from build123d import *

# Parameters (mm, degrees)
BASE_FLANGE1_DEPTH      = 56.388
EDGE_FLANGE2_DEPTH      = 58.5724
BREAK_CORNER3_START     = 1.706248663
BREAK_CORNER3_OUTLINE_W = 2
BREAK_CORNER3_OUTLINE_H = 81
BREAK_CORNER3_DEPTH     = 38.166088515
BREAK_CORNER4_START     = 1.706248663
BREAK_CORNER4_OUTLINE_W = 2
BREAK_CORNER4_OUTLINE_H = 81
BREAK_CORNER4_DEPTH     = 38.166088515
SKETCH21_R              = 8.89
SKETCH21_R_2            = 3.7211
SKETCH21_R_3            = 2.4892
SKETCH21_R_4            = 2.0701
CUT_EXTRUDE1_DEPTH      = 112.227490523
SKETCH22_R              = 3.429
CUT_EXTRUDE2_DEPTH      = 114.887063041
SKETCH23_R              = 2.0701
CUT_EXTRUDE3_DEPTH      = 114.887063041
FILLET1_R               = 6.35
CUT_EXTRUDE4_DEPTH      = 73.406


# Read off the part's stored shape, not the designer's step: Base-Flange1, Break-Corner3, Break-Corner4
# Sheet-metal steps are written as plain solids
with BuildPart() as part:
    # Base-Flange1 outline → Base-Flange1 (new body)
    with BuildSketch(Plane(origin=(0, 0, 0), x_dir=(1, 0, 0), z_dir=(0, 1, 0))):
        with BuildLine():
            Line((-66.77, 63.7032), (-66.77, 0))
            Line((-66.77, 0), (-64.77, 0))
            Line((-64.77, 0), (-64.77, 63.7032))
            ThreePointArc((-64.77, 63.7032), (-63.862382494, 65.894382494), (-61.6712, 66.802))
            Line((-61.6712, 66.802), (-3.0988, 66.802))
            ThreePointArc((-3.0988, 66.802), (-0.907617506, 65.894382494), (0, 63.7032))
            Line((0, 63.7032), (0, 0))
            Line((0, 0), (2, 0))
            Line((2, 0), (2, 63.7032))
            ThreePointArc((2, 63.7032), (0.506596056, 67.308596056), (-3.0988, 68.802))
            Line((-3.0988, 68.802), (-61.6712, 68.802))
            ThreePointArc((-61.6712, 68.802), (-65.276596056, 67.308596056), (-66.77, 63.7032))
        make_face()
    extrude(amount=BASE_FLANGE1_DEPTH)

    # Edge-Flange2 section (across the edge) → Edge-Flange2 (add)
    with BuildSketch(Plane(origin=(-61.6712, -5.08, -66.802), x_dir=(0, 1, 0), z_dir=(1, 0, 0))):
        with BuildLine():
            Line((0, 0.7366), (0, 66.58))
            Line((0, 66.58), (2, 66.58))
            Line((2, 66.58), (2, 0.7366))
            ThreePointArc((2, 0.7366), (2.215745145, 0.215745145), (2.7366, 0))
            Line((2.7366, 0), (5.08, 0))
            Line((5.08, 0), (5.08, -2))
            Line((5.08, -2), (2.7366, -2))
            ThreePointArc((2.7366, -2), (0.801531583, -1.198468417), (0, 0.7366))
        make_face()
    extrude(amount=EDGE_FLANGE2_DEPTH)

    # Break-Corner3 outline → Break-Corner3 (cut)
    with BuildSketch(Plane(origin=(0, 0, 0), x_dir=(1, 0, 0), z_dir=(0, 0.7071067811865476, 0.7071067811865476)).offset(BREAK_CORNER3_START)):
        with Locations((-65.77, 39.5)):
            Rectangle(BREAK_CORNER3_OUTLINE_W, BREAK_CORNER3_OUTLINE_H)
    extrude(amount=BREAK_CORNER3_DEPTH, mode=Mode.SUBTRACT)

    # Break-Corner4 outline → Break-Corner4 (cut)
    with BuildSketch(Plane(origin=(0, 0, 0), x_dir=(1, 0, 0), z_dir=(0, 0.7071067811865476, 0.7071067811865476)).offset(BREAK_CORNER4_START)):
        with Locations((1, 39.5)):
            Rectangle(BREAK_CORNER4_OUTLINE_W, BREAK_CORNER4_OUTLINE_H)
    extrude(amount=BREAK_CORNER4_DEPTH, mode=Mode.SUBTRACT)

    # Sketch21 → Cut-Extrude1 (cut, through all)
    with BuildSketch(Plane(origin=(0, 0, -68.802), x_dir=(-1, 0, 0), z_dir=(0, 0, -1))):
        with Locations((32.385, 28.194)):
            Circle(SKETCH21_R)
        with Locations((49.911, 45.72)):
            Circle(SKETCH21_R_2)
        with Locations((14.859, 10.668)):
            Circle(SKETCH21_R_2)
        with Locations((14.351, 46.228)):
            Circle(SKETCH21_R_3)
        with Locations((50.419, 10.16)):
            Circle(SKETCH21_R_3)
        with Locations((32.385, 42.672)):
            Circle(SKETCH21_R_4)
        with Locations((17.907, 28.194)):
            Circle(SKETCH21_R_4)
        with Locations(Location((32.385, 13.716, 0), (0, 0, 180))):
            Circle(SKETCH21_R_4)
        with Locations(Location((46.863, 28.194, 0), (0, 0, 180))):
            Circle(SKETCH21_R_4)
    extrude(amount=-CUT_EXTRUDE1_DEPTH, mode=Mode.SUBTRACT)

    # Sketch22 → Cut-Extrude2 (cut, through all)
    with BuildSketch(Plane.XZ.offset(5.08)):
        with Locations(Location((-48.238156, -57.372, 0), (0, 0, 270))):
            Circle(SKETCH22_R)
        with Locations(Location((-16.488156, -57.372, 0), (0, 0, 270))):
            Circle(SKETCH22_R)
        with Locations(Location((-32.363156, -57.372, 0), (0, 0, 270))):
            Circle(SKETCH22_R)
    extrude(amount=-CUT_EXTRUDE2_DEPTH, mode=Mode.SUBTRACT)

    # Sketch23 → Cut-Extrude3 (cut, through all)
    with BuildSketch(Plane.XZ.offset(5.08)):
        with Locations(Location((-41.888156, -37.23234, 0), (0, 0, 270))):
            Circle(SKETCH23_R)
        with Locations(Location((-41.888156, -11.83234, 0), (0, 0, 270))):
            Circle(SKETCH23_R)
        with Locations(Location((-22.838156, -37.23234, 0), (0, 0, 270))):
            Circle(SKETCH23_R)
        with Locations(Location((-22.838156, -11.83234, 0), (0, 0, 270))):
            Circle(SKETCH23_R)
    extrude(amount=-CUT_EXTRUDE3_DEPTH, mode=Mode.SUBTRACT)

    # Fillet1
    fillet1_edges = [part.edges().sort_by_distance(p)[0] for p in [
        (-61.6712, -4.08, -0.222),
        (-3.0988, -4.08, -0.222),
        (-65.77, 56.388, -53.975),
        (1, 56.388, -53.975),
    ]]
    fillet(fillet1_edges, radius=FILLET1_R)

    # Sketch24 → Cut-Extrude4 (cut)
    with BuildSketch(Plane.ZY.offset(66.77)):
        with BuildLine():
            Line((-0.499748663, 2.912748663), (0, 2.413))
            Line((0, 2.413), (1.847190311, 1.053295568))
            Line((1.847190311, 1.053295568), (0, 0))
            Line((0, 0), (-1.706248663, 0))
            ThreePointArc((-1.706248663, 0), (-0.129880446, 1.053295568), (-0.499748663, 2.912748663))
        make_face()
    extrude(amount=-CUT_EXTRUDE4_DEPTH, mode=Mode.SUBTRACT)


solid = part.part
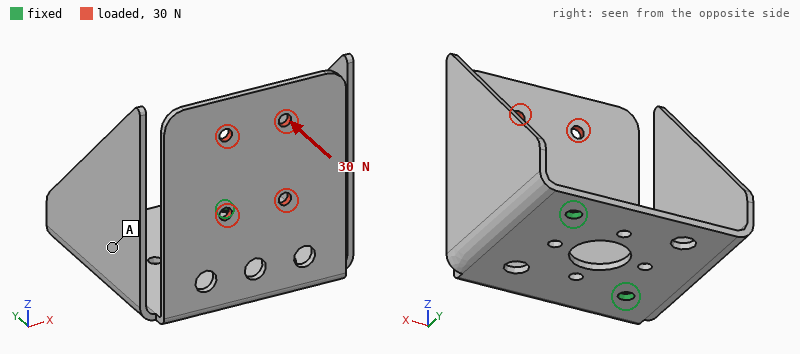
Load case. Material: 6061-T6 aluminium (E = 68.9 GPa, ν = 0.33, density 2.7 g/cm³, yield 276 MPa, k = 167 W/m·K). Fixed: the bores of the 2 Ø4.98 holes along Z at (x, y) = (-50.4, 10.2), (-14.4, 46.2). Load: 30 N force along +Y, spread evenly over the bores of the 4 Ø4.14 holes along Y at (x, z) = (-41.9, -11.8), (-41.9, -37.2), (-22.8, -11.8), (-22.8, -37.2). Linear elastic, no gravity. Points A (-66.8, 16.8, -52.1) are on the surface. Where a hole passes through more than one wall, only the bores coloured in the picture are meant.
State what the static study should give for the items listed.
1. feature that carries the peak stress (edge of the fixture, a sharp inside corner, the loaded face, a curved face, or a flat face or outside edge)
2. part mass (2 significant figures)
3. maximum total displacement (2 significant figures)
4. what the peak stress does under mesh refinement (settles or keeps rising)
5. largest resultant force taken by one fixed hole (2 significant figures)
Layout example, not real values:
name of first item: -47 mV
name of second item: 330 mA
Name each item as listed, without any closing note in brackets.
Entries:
feature that carries the peak stress: a sharp inside corner
part mass: 64 g
maximum total displacement: 1.1 mm
what the peak stress does under mesh refinement: keeps rising
largest resultant force taken by one fixed hole: 18 N
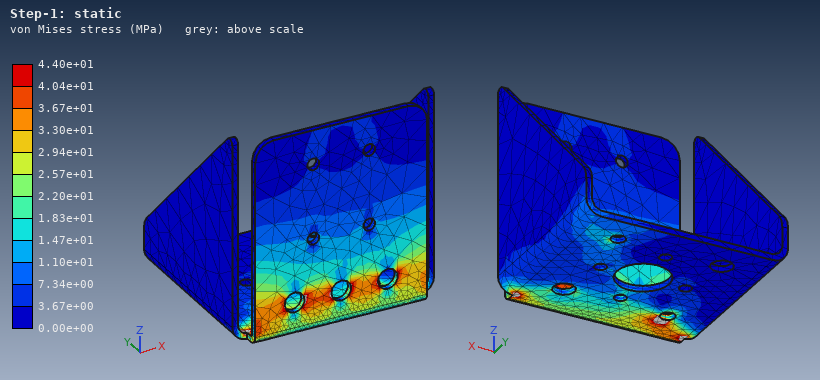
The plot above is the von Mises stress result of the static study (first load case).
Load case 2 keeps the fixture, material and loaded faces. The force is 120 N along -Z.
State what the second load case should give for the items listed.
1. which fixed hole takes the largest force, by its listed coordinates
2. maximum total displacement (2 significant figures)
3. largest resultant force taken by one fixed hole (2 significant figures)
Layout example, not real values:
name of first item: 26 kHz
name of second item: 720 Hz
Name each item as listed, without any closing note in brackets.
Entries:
which fixed hole takes the largest force, by its listed coordinates: (-50.4, 10.2)
maximum total displacement: 0.65 mm
largest resultant force taken by one fixed hole: 100 N
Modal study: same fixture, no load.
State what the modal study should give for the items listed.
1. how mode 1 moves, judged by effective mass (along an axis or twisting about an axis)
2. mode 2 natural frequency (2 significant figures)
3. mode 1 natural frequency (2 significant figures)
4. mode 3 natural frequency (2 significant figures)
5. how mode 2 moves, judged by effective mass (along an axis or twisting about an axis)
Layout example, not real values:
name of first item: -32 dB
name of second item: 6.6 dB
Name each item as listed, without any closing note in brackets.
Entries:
how mode 1 moves, judged by effective mass: along Y
mode 2 natural frequency: 380 Hz
mode 1 natural frequency: 250 Hz
mode 3 natural frequency: 420 Hz
how mode 2 moves, judged by effective mass: along X
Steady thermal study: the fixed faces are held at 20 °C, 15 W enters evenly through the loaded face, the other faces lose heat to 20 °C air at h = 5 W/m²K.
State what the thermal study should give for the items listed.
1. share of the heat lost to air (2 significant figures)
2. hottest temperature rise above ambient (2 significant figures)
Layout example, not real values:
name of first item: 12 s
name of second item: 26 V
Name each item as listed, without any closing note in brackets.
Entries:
share of the heat lost to air: 14 %
hottest temperature rise above ambient: 53 K
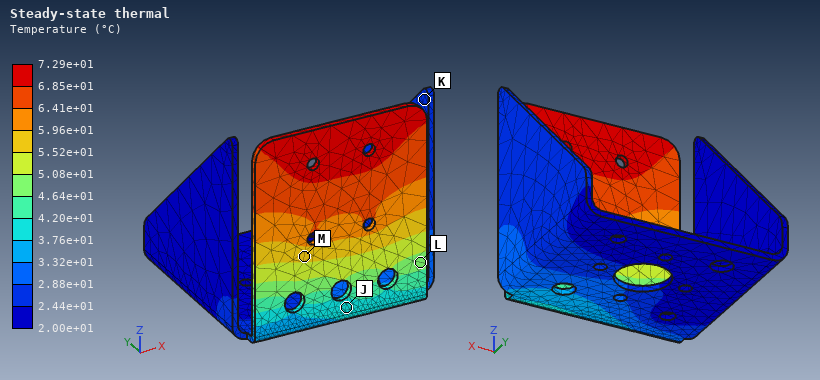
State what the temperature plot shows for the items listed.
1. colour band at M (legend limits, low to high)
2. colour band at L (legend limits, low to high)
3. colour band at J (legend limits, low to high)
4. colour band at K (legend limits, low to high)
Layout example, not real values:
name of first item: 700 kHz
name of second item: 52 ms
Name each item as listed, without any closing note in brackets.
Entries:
colour band at M: 5.52e+01 to 5.96e+01 °C
colour band at L: 4.64e+01 to 5.08e+01 °C
colour band at J: 3.76e+01 to 4.20e+01 °C
colour band at K: 2.44e+01 to 2.88e+01 °C
